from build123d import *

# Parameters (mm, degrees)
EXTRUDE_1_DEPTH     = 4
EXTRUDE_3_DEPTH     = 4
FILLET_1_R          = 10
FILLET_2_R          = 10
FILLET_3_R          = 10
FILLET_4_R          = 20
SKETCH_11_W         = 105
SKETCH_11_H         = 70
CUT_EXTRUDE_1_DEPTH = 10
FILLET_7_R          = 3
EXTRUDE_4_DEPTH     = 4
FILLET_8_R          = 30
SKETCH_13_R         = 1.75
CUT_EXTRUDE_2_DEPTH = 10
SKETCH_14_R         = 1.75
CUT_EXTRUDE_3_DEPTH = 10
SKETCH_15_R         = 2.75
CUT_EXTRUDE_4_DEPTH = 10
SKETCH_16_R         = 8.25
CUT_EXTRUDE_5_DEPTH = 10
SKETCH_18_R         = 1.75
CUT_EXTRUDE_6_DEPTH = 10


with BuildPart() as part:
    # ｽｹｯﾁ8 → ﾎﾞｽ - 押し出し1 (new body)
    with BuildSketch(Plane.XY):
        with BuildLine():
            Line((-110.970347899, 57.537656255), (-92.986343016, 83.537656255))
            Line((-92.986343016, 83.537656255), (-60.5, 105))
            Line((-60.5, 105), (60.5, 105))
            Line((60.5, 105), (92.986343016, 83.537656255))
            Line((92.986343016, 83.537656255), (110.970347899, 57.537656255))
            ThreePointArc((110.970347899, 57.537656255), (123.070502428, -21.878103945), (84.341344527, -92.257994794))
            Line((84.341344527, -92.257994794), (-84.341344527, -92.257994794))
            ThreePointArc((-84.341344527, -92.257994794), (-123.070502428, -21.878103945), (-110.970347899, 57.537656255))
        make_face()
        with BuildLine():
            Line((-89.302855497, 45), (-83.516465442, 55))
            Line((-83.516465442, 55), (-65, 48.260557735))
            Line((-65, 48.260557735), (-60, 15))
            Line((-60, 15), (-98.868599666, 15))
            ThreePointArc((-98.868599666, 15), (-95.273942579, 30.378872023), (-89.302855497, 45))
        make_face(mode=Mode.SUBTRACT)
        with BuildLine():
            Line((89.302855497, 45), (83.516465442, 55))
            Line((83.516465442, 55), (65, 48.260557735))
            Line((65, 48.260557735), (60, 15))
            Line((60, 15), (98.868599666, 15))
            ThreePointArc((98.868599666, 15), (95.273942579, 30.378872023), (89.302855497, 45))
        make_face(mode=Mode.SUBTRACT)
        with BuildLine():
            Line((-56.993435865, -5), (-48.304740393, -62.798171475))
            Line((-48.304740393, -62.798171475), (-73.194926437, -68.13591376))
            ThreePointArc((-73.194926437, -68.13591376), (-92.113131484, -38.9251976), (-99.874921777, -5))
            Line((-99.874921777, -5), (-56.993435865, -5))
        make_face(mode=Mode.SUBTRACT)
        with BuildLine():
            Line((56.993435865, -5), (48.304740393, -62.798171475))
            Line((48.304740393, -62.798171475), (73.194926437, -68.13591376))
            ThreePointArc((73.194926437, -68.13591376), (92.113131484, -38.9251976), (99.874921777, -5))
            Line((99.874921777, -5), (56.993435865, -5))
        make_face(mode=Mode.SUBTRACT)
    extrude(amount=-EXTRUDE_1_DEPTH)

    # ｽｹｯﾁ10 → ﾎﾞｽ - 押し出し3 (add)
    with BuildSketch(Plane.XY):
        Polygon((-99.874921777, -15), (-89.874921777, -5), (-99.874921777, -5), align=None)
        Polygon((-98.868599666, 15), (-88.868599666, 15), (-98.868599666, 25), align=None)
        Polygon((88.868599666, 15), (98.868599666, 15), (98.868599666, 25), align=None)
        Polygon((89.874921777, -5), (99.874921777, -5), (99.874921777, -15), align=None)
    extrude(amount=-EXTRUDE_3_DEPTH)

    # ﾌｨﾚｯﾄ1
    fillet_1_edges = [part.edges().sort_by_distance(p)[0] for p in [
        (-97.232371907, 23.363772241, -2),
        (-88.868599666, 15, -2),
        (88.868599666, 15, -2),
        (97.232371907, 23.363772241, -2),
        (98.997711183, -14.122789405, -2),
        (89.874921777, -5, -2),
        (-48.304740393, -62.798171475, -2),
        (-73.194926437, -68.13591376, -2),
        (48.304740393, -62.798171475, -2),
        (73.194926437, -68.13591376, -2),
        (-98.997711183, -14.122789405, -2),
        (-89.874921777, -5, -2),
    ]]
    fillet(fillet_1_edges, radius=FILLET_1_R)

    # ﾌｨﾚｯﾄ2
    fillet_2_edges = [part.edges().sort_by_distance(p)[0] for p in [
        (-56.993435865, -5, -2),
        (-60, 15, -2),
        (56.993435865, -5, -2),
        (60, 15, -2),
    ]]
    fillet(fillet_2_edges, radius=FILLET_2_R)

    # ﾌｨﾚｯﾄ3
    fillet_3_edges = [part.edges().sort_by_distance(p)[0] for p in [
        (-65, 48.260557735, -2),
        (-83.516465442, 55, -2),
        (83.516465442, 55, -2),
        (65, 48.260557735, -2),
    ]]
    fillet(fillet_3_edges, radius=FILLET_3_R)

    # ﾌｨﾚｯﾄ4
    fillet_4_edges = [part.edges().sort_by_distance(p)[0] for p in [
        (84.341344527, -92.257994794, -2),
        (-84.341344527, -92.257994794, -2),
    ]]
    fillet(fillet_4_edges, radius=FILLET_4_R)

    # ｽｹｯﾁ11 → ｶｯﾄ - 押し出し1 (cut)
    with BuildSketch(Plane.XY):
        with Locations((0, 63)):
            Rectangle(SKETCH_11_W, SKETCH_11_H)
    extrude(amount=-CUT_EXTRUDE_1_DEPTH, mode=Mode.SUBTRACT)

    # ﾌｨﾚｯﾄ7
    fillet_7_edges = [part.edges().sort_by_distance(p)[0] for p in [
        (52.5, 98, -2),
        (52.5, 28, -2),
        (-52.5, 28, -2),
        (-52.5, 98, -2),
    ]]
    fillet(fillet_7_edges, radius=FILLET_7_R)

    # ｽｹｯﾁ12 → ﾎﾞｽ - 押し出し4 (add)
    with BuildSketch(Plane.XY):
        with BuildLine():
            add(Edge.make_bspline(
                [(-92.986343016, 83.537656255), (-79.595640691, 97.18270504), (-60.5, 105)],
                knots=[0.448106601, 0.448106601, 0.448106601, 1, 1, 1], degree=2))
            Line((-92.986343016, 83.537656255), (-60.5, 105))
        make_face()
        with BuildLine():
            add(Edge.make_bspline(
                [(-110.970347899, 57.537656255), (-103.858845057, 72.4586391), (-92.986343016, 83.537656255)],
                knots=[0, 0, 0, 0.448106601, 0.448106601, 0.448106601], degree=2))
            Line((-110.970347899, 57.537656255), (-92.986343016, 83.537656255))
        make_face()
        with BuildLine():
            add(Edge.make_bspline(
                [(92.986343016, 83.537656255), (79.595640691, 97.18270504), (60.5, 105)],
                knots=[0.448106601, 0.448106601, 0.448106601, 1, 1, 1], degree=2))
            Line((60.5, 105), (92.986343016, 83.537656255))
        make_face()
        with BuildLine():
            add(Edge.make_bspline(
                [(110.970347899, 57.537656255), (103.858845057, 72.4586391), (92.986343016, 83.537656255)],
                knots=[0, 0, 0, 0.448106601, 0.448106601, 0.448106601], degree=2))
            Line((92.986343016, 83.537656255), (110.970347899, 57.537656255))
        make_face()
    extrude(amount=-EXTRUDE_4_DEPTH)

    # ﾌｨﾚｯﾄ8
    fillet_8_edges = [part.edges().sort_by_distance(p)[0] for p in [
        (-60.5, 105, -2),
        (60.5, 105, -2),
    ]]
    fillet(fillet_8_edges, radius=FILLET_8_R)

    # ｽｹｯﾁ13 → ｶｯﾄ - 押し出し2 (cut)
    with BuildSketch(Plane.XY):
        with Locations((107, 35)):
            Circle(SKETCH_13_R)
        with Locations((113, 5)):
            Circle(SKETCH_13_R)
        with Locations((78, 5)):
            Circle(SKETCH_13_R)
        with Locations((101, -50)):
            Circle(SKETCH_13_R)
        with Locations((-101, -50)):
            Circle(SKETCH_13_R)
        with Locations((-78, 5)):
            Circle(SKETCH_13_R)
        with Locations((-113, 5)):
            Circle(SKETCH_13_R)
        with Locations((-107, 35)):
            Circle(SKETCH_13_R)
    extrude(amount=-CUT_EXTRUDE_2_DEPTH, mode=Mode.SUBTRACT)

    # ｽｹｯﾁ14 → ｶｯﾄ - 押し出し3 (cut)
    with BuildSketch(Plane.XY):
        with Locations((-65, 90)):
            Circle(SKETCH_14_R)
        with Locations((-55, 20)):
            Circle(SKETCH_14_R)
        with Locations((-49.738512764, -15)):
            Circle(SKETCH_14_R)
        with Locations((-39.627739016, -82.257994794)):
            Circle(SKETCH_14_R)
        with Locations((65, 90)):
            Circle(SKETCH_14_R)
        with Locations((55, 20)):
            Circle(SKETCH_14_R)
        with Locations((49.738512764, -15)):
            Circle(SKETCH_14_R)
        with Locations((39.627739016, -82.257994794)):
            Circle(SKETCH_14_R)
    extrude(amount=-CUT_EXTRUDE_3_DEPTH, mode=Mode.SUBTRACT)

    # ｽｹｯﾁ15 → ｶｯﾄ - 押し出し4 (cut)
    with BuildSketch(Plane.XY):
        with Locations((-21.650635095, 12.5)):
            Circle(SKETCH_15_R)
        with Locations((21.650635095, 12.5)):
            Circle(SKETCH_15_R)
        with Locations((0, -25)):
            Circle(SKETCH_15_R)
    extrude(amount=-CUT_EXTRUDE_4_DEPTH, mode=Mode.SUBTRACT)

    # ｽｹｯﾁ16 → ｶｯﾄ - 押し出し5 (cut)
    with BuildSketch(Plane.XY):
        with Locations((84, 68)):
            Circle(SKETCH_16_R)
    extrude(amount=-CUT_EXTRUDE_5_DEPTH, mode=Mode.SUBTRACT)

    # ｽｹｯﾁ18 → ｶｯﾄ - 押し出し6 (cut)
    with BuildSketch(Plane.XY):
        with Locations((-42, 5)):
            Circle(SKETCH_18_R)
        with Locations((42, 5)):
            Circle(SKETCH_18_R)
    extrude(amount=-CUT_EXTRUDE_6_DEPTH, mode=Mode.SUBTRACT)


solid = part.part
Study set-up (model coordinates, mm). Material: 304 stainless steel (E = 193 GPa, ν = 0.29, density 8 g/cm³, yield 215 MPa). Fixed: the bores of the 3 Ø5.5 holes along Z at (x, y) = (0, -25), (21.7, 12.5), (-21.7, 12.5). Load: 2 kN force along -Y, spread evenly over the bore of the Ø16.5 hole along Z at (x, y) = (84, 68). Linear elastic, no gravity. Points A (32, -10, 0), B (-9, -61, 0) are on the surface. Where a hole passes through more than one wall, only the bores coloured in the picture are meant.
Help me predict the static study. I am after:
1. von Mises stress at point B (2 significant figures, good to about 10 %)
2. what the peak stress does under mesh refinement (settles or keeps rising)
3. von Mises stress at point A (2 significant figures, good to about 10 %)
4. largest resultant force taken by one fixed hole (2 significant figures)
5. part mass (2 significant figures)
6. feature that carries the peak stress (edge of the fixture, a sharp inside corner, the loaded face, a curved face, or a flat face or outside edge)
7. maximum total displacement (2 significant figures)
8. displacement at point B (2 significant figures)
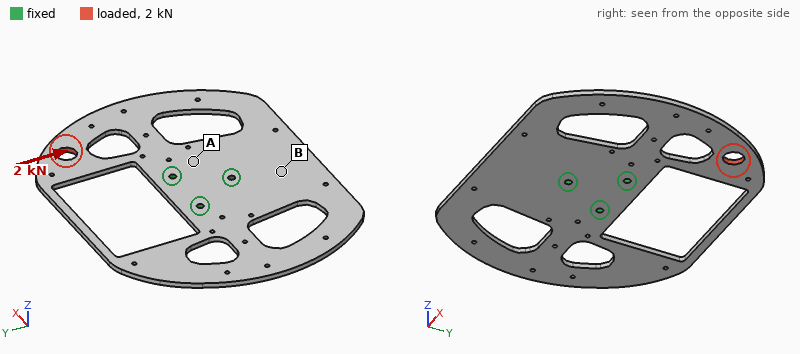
5.6 MPa
keeps rising
20 MPa
2.7 kN
930 g
edge of the fixture
35 µm
6.6 µm
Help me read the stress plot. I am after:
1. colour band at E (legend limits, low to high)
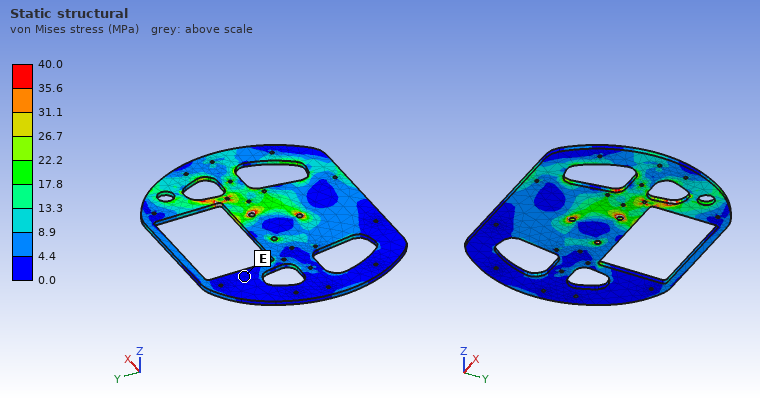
0.0 to 4.4 MPa
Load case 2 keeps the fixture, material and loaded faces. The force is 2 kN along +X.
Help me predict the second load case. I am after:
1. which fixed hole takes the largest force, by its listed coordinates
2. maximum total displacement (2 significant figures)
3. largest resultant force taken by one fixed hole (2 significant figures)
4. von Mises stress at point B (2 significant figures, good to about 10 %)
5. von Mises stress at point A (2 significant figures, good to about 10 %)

(21.7, 12.5)
56 µm
2.4 kN
7.4 MPa
11 MPa
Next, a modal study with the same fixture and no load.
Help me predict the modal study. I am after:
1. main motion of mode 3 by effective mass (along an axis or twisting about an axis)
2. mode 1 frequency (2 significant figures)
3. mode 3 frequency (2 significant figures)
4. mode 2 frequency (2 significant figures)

along Z
210 Hz
270 Hz
220 Hz
